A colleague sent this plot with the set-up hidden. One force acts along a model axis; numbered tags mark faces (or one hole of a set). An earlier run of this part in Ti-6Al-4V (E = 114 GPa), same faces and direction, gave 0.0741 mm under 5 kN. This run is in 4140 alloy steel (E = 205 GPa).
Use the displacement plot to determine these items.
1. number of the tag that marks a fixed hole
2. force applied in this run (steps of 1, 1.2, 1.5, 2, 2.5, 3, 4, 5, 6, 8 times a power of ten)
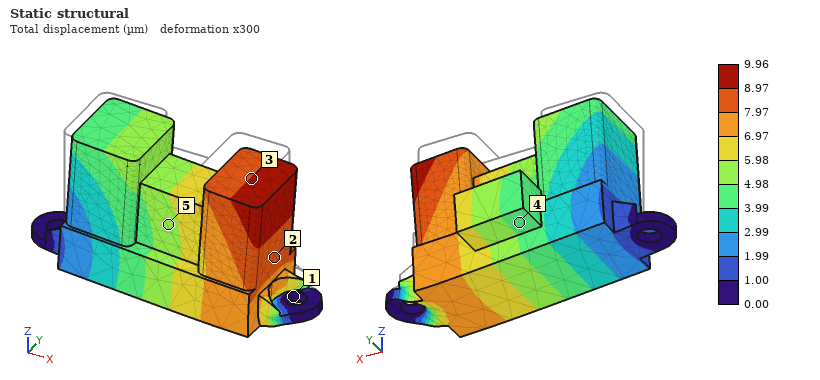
1
1.2 kN
